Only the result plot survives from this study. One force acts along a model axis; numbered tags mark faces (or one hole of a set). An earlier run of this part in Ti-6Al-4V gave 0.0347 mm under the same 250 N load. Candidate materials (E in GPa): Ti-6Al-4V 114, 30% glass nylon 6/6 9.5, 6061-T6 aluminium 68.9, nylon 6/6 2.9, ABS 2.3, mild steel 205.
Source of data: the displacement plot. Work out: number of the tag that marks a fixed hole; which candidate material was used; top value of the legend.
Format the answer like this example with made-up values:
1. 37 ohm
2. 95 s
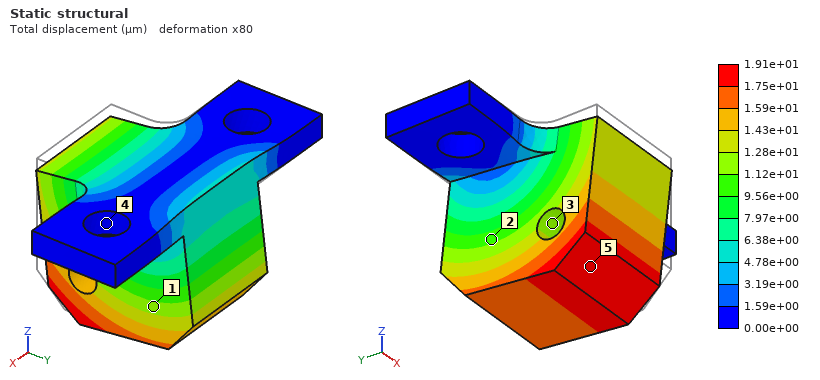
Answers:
1. 4
2. mild steel
3. 1.91e+01 µm
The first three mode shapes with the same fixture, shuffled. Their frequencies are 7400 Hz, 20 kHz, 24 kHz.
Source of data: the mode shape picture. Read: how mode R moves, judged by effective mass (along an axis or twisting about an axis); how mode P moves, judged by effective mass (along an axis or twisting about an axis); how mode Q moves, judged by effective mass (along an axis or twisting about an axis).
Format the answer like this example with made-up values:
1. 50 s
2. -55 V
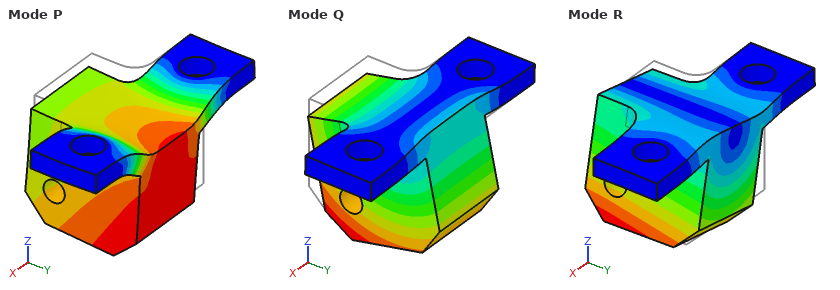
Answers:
1. along X
2. along Z
3. along Y
